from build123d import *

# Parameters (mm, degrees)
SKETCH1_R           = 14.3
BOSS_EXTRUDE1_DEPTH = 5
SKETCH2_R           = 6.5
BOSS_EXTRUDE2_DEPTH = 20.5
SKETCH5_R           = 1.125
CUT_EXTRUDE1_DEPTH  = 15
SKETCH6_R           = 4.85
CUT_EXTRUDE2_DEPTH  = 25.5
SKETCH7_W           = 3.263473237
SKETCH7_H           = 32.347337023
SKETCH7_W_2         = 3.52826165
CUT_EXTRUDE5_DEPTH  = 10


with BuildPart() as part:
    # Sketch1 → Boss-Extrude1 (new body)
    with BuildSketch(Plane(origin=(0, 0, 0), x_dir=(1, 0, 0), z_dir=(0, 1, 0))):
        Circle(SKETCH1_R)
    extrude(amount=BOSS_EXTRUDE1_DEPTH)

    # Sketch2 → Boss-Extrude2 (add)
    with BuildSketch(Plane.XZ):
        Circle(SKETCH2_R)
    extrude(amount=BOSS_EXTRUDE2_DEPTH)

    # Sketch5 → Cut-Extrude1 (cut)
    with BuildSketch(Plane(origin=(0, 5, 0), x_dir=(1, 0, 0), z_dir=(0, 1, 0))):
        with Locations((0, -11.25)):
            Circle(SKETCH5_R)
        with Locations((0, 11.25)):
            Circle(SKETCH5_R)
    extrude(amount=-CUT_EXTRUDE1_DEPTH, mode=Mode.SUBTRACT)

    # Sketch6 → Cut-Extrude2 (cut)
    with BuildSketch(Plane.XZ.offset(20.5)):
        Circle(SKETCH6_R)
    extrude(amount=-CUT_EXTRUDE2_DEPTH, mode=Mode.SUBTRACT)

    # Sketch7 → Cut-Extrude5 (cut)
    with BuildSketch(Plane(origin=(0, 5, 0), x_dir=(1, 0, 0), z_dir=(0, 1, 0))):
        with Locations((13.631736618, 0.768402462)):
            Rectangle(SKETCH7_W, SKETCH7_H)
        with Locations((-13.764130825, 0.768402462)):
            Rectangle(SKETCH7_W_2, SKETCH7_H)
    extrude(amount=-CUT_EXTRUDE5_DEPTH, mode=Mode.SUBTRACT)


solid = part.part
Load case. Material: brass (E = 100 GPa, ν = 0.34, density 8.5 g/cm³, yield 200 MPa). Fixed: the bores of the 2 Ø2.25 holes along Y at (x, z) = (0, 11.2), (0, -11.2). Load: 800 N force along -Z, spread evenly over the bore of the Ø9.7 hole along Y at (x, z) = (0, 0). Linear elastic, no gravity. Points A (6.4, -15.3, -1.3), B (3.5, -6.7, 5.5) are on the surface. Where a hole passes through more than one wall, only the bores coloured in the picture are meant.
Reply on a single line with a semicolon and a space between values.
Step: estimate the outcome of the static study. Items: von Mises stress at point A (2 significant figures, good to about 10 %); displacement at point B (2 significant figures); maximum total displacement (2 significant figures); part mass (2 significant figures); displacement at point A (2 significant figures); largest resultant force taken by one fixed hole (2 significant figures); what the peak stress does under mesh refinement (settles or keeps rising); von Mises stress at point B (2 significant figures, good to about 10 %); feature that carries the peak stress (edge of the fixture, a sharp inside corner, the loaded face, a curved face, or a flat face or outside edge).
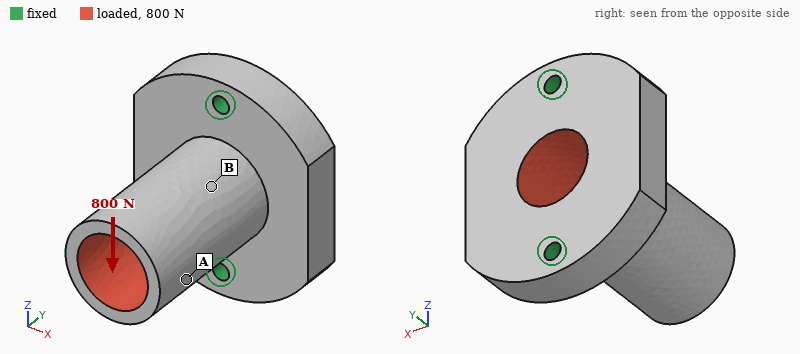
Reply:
8.6 MPa; 9.3 µm; 23 µm; 32 g; 17 µm; 600 N; keeps rising; 19 MPa; edge of the fixture
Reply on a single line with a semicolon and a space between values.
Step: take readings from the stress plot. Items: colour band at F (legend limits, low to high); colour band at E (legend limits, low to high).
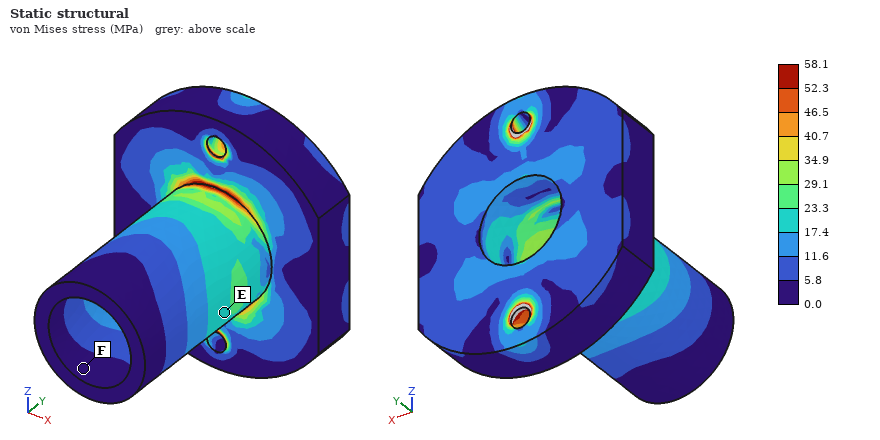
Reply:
0.0 to 5.8 MPa; 17.4 to 23.3 MPa
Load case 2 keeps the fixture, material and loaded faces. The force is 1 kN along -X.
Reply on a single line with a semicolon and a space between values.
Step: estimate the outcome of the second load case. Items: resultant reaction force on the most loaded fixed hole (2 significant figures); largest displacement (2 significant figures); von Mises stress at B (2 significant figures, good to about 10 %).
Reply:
500 N; 70 µm; 26 MPa
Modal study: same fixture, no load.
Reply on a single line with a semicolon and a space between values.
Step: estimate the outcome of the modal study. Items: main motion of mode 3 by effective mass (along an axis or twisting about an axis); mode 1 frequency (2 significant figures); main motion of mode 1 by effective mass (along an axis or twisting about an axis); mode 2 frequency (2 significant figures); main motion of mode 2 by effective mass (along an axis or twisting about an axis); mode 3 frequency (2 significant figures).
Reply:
along Y; 5800 Hz; along X; 9800 Hz; along Z; 14 kHz
